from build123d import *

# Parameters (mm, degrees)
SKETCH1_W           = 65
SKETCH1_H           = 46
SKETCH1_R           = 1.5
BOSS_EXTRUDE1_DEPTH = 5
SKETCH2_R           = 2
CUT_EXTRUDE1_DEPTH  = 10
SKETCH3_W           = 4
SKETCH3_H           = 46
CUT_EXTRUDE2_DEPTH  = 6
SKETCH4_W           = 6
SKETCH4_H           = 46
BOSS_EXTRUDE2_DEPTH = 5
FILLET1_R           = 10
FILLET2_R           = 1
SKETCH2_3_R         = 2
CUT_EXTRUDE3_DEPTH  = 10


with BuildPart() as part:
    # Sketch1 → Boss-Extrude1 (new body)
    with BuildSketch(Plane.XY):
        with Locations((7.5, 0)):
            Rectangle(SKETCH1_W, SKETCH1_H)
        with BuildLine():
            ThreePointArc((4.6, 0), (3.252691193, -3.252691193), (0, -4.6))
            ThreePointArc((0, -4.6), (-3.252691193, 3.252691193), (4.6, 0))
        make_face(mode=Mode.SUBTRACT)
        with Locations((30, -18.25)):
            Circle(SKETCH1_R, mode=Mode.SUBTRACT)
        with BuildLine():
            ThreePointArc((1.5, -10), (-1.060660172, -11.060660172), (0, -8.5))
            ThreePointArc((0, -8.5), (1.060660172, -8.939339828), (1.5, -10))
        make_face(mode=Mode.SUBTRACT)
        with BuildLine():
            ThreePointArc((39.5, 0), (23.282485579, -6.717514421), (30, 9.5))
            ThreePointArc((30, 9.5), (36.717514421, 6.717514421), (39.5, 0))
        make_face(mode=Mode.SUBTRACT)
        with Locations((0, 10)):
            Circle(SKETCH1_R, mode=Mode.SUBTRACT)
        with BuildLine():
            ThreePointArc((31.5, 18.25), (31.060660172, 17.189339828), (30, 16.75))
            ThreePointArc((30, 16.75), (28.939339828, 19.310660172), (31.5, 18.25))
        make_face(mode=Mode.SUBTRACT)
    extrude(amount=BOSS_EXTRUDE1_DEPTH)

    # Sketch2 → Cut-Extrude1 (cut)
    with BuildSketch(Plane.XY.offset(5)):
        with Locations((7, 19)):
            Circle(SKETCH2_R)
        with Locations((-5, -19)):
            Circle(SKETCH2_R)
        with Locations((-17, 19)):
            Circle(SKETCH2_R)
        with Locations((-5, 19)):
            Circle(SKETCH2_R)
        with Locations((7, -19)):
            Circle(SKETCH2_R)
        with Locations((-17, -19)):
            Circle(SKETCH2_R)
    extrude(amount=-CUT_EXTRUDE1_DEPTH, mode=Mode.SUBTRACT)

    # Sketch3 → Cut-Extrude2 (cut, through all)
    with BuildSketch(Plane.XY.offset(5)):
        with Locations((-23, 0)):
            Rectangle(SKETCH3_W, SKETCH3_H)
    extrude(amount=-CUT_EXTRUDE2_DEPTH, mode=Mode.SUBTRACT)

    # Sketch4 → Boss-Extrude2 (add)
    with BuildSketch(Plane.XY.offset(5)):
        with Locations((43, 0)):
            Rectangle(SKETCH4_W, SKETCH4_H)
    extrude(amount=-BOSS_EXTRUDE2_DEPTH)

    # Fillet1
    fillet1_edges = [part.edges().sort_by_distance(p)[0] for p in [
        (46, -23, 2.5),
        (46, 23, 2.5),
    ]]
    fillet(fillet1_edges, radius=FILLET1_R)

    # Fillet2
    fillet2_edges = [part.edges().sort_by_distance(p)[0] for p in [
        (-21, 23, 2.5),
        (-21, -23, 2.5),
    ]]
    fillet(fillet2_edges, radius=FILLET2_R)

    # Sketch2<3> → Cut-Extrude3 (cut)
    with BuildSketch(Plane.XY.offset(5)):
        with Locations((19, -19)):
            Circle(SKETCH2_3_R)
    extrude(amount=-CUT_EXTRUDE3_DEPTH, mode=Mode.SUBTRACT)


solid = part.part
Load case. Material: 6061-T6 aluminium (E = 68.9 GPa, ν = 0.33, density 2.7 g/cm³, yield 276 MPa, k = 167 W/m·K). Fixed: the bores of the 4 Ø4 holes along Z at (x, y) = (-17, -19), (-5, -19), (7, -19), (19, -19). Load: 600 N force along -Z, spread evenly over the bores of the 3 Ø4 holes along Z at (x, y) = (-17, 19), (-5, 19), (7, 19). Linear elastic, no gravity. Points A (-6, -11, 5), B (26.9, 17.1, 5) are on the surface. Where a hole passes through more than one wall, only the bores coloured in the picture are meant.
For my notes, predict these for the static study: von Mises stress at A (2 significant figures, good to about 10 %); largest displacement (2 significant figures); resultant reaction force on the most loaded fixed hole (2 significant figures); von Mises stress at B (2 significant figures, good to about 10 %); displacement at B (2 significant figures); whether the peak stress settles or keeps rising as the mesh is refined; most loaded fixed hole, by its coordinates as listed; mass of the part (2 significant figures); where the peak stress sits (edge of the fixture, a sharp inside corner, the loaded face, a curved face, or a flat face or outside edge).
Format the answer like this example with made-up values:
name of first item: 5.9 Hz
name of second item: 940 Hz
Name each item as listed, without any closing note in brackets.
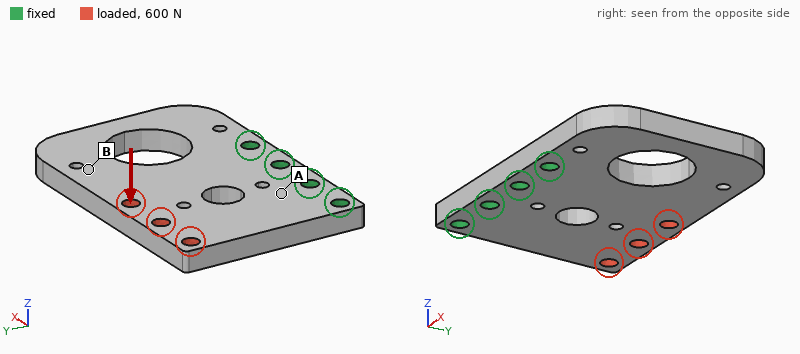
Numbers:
von Mises stress at A: 93 MPa
largest displacement: 0.43 mm
resultant reaction force on the most loaded fixed hole: 240 N
von Mises stress at B: 25 MPa
displacement at B: 0.22 mm
whether the peak stress settles or keeps rising as the mesh is refined: keeps rising
most loaded fixed hole, by its coordinates as listed: (-5, -19)
mass of the part: 35 g
where the peak stress sits: edge of the fixture
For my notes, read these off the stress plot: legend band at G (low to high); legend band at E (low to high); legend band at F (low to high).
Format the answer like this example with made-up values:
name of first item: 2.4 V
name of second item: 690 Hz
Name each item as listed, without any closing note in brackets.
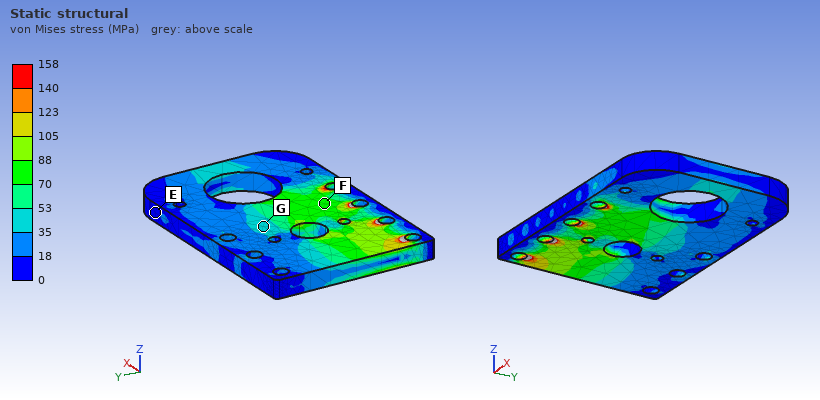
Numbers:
legend band at G: 35 to 53 MPa
legend band at E: 0 to 18 MPa
legend band at F: 70 to 88 MPa
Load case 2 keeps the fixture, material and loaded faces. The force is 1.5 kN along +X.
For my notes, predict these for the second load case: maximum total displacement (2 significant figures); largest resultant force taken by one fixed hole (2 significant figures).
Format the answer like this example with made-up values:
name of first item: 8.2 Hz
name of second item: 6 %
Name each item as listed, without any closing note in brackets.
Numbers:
maximum total displacement: 32 µm
largest resultant force taken by one fixed hole: 1.5 kN
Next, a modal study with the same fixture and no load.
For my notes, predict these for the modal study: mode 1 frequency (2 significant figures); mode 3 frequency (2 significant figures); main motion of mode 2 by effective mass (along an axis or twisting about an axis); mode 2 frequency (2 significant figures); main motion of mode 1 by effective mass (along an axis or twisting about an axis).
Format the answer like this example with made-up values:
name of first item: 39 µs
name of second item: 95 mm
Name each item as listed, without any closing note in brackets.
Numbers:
mode 1 frequency: 2000 Hz
mode 3 frequency: 6000 Hz
main motion of mode 2 by effective mass: twisting about Y
mode 2 frequency: 3200 Hz
main motion of mode 1 by effective mass: along Z
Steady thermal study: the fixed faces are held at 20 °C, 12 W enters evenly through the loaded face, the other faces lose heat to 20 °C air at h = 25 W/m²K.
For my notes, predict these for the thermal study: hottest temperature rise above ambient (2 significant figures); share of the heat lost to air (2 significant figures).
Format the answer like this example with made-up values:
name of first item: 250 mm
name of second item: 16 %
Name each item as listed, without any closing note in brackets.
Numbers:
hottest temperature rise above ambient: 16 K
share of the heat lost to air: 7.6 %
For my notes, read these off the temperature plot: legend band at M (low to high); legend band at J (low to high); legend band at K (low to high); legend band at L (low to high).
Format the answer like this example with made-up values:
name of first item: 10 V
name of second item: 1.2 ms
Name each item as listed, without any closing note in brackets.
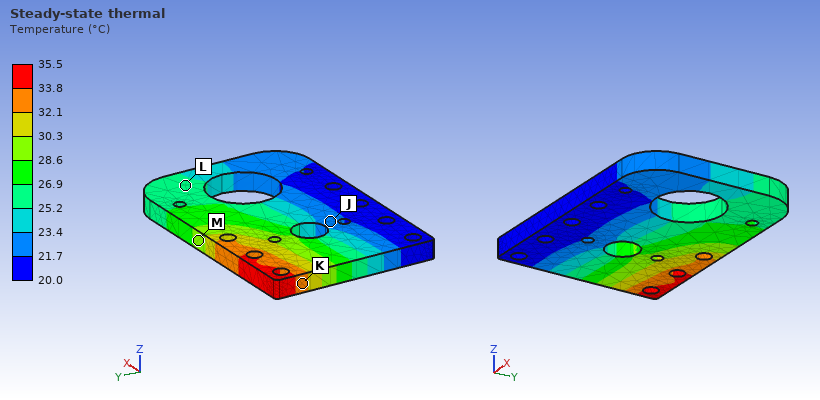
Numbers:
legend band at M: 28.6 to 30.3 °C
legend band at J: 21.7 to 23.4 °C
legend band at K: 32.1 to 33.8 °C
legend band at L: 25.2 to 26.9 °C
